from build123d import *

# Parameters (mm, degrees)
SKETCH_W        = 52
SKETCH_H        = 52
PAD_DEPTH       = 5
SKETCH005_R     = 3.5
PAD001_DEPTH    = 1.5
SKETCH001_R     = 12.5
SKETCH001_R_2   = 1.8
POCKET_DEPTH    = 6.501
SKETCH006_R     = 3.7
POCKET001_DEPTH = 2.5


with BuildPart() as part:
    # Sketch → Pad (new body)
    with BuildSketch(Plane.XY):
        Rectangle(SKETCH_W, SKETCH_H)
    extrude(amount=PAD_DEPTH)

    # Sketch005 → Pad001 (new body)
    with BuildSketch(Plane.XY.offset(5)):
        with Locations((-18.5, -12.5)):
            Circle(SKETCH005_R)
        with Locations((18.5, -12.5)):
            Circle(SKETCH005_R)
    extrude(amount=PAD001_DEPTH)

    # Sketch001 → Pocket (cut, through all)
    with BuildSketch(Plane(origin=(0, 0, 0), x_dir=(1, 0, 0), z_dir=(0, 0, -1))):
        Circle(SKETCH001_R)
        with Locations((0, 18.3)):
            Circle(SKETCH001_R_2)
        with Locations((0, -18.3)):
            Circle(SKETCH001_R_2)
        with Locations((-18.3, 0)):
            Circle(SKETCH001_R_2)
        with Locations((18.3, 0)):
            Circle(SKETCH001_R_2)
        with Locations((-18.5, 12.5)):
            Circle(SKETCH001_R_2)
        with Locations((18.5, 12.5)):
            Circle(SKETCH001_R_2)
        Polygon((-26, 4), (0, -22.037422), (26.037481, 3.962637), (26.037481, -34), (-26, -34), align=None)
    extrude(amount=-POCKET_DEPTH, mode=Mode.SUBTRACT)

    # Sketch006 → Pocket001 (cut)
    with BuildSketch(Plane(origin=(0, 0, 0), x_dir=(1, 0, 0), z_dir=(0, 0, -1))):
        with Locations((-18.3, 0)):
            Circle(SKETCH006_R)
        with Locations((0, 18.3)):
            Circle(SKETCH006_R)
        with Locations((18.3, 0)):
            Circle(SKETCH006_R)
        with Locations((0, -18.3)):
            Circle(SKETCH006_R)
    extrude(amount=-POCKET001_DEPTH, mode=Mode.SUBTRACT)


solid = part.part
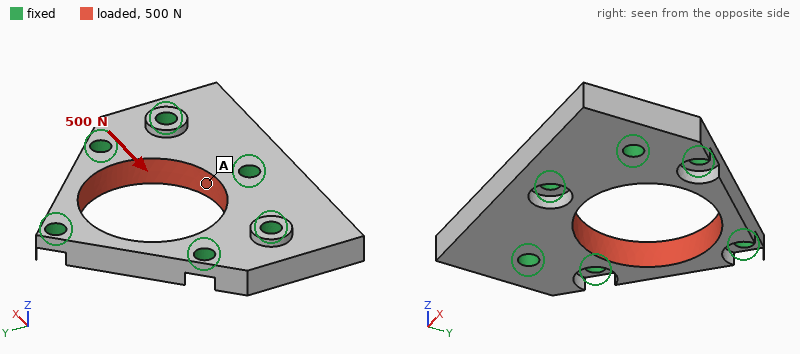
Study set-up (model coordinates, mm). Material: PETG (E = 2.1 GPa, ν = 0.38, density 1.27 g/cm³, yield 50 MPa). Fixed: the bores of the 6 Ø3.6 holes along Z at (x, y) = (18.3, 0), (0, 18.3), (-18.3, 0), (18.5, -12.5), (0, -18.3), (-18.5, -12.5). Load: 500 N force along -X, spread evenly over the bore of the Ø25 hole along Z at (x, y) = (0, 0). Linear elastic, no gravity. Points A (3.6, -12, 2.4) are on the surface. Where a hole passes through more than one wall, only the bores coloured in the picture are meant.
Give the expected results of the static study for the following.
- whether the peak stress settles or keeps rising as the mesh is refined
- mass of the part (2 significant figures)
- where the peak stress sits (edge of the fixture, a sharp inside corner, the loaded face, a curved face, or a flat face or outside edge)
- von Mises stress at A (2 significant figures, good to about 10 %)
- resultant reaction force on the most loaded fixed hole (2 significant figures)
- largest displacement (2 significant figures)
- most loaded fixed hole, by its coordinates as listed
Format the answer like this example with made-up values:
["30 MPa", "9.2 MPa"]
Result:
["keeps rising", "7.8 g", "edge of the fixture", "2.2 MPa", "140 N", "91 µm", "(0, 18.3)"]
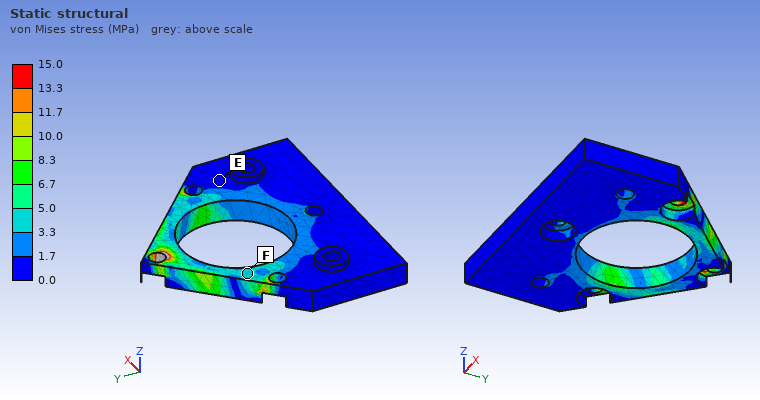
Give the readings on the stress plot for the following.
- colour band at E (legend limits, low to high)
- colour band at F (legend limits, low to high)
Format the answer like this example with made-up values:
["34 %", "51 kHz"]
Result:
["0.0 to 1.7 MPa", "3.3 to 5.0 MPa"]
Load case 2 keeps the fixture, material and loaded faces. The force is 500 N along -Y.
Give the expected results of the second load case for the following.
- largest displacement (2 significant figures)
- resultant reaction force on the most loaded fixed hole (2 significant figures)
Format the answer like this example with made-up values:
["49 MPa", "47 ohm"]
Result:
["53 µm", "100 N"]
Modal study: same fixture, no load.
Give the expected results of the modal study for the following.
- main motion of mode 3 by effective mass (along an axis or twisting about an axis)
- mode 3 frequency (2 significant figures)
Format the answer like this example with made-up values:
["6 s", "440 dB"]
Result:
["along Z", "5900 Hz"]
